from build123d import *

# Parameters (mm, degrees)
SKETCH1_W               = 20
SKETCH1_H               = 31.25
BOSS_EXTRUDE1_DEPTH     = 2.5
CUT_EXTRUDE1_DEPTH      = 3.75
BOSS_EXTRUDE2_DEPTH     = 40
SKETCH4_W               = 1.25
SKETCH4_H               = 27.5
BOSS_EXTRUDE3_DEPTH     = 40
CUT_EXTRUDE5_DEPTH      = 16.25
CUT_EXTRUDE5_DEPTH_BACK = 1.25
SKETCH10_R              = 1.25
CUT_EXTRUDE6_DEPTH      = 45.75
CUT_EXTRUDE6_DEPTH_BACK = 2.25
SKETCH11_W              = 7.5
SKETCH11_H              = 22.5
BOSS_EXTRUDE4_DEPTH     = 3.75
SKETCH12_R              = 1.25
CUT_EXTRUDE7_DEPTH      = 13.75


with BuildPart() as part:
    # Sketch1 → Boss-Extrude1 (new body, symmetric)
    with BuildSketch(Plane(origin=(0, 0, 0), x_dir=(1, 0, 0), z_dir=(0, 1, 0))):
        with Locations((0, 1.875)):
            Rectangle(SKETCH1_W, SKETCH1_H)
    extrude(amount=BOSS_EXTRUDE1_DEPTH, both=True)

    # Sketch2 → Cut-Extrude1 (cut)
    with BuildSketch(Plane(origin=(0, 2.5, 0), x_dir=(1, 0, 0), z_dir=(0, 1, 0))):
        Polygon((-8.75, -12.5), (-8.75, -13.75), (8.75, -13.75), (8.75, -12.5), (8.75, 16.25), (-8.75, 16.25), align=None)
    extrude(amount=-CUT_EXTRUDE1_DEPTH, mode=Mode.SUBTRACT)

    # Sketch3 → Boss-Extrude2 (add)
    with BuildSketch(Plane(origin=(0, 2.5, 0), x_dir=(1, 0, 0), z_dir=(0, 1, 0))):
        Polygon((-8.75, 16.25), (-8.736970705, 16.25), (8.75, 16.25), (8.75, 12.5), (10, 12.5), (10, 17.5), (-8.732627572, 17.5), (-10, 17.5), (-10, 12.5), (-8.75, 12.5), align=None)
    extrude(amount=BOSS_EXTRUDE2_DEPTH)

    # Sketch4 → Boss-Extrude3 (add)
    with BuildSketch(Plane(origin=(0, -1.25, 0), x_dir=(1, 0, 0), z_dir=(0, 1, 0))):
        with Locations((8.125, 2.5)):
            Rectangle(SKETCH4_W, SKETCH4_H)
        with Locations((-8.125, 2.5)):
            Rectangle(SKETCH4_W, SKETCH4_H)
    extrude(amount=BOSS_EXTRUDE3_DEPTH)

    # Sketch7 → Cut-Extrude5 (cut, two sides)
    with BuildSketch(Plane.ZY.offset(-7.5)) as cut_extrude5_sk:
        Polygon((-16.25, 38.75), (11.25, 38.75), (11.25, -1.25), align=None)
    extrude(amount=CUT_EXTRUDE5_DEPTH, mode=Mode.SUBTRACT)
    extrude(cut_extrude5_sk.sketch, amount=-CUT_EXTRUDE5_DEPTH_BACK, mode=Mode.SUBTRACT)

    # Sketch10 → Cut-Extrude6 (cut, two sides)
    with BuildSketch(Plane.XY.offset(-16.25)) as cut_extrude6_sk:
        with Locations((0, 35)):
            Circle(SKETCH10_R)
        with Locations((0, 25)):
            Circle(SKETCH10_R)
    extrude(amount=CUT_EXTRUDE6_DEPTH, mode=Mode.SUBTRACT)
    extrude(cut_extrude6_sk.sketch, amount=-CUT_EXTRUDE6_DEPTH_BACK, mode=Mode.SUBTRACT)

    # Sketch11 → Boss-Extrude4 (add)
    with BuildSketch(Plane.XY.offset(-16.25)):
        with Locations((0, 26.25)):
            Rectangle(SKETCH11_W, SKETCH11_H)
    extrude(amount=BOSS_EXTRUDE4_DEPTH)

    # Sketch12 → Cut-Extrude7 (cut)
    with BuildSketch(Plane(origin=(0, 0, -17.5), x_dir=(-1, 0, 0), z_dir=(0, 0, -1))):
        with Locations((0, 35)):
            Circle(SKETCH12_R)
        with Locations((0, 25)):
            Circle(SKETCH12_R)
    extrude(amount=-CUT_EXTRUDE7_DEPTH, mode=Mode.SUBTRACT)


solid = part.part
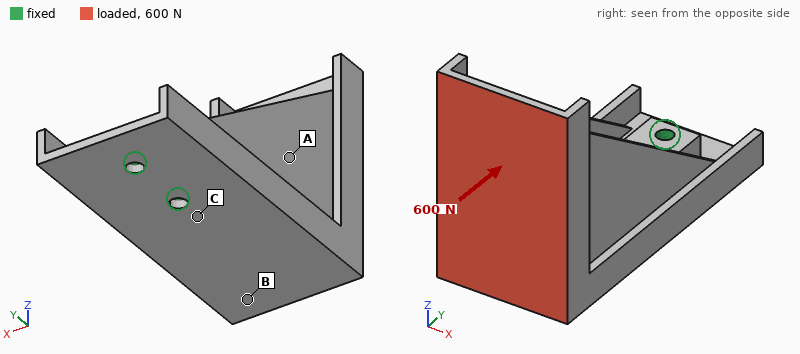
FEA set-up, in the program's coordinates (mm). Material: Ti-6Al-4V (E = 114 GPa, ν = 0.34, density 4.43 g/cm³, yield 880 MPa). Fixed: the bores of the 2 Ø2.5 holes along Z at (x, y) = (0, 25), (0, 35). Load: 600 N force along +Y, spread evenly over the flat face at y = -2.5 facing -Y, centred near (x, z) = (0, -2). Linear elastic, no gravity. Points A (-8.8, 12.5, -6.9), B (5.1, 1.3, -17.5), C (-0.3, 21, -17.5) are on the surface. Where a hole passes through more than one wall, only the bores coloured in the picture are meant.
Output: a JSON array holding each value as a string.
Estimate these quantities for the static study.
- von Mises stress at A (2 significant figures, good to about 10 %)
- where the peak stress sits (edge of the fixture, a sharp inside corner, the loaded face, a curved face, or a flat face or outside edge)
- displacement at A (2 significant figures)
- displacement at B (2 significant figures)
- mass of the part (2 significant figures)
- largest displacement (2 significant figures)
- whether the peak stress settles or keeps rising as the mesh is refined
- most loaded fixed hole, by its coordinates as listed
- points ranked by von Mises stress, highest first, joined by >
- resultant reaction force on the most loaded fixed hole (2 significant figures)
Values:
["29 MPa", "edge of the fixture", "0.061 mm", "0.096 mm", "20 g", "0.20 mm", "keeps rising", "(0, 25)", "C > A > B", "690 N"]
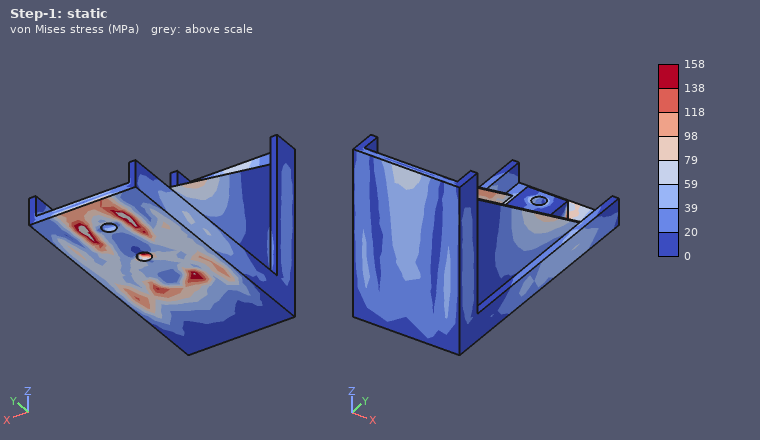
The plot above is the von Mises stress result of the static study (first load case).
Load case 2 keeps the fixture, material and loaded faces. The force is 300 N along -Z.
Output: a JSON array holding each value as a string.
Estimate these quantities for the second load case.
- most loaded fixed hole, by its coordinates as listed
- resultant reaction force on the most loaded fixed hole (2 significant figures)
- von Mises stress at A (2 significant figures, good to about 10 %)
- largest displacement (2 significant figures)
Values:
["(0, 25)", "760 N", "23 MPa", "0.18 mm"]
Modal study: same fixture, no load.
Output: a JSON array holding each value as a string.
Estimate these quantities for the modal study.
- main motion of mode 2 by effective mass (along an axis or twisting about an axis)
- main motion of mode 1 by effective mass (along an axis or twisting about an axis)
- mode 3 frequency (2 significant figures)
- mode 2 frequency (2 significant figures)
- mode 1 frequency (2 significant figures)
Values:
["along Z", "along X", "6200 Hz", "2500 Hz", "1500 Hz"]
